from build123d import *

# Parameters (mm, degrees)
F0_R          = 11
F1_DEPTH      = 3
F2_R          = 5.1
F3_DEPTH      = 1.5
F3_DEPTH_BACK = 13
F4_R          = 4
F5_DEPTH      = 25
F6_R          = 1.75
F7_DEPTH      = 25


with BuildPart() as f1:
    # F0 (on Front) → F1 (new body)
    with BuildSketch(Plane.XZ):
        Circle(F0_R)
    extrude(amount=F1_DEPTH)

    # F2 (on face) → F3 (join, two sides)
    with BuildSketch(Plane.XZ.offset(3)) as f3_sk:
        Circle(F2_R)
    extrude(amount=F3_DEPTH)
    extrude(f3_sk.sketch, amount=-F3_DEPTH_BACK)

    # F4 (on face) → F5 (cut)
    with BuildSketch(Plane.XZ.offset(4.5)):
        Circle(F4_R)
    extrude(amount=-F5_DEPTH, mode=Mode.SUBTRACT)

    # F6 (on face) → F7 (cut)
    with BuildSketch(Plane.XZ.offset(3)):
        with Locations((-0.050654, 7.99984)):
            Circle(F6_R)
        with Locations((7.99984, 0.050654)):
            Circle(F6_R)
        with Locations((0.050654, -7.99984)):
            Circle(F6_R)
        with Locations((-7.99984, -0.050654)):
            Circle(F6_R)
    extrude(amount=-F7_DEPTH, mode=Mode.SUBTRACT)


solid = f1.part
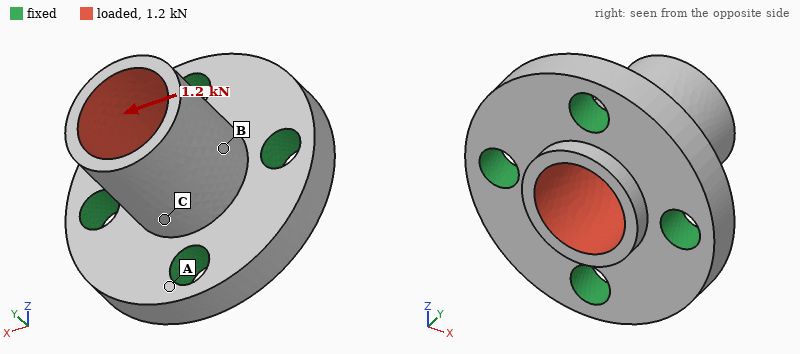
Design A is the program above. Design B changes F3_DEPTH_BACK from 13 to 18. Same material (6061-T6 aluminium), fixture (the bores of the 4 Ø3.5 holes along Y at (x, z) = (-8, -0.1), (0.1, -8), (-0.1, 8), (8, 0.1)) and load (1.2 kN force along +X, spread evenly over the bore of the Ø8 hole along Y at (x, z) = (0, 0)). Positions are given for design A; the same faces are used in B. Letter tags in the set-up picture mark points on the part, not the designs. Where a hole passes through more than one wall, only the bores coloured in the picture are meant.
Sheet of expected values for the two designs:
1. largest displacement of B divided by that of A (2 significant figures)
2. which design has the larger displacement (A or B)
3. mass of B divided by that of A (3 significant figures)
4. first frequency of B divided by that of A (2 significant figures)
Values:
2.2
B
1.13
0.59
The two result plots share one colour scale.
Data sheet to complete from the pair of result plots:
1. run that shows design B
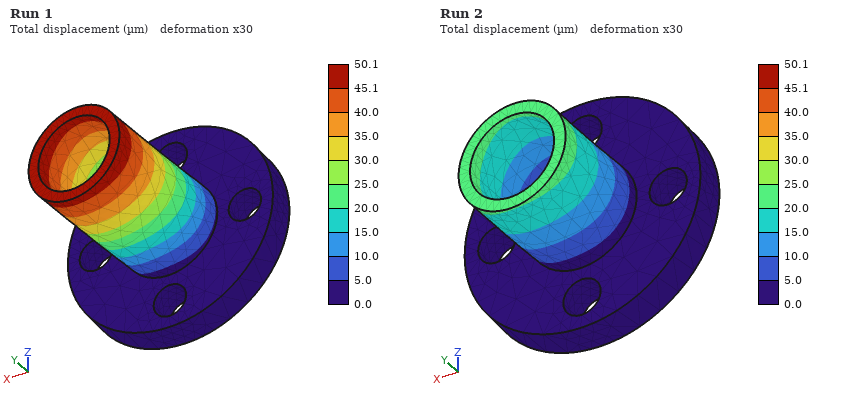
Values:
Run 1
